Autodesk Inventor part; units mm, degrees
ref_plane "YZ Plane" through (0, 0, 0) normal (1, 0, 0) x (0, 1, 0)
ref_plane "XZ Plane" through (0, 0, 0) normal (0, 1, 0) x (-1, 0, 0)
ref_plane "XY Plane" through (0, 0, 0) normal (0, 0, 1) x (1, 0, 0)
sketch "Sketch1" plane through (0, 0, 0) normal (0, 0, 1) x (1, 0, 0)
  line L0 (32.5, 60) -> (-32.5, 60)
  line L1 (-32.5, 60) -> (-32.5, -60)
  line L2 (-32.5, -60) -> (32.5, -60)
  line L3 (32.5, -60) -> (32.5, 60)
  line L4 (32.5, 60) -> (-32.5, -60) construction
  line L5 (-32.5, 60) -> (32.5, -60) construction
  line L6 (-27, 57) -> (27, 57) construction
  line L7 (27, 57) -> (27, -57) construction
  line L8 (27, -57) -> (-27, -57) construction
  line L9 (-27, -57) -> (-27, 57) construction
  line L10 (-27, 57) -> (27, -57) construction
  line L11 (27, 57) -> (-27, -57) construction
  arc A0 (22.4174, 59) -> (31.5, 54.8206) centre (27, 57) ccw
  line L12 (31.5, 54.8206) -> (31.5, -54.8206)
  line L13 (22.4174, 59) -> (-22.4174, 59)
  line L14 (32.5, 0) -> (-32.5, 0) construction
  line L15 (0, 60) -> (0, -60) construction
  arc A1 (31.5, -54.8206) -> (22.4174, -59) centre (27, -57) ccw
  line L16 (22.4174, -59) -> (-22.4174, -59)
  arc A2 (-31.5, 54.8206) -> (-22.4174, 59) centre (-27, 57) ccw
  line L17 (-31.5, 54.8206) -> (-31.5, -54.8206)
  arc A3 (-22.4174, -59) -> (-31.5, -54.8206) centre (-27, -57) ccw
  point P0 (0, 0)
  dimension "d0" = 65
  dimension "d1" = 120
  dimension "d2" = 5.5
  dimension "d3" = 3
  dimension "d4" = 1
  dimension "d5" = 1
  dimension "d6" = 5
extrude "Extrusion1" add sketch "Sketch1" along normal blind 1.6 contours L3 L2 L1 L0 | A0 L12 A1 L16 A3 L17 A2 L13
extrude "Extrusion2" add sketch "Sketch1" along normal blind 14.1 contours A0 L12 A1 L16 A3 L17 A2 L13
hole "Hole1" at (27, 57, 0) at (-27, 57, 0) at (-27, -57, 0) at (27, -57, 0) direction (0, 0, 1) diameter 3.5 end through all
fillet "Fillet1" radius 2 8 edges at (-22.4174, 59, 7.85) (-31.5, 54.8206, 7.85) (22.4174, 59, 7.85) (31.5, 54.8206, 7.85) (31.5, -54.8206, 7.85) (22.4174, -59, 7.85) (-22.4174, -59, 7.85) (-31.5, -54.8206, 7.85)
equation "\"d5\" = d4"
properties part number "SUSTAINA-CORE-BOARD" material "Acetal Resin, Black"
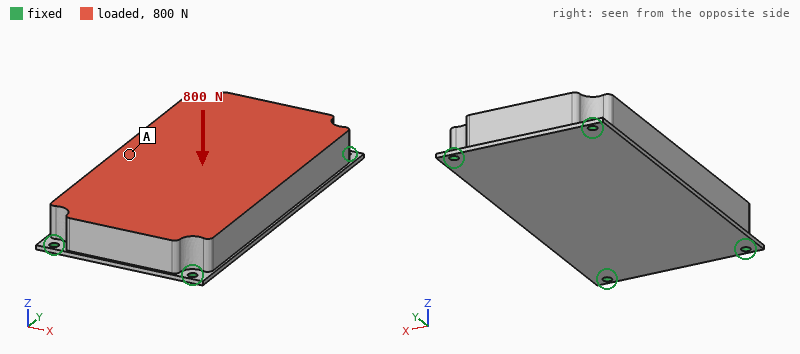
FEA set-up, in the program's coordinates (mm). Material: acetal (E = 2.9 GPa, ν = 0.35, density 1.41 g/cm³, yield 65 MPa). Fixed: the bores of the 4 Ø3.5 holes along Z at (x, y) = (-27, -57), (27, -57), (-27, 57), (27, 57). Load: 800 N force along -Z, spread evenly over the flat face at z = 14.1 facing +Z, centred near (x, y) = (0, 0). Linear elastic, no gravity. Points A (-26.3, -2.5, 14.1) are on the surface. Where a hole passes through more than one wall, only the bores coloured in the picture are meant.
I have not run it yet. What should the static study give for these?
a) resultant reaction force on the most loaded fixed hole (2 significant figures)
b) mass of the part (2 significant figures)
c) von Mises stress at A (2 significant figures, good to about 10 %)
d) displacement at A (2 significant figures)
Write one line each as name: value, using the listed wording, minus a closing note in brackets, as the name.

resultant reaction force on the most loaded fixed hole: 310 N
mass of the part: 140 g
von Mises stress at A: 4.1 MPa
displacement at A: 0.36 mm
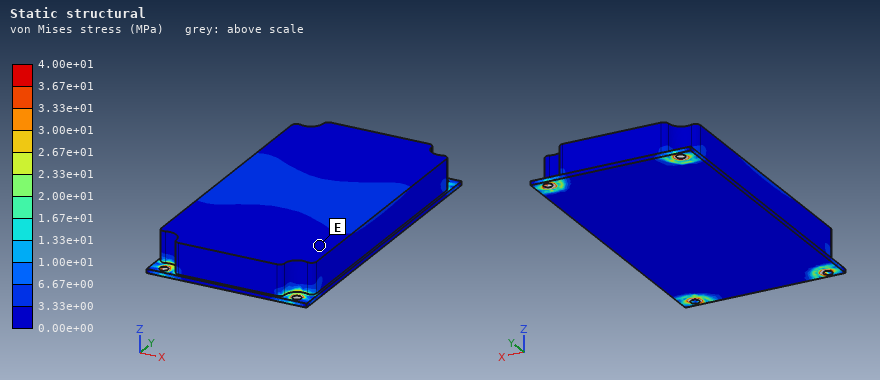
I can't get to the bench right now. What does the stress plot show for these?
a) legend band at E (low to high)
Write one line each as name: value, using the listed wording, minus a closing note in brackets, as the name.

legend band at E: 0.00e+00 to 3.33e+00 MPa
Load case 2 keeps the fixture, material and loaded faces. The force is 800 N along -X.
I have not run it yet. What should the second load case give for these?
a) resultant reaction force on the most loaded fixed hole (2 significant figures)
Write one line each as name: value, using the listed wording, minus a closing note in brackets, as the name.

resultant reaction force on the most loaded fixed hole: 250 N
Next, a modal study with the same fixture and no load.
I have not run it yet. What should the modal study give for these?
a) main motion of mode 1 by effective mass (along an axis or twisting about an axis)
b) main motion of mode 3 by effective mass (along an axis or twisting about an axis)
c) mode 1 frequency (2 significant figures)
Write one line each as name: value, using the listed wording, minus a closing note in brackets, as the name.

main motion of mode 1 by effective mass: along Z
main motion of mode 3 by effective mass: twisting about X
mode 1 frequency: 700 Hz
